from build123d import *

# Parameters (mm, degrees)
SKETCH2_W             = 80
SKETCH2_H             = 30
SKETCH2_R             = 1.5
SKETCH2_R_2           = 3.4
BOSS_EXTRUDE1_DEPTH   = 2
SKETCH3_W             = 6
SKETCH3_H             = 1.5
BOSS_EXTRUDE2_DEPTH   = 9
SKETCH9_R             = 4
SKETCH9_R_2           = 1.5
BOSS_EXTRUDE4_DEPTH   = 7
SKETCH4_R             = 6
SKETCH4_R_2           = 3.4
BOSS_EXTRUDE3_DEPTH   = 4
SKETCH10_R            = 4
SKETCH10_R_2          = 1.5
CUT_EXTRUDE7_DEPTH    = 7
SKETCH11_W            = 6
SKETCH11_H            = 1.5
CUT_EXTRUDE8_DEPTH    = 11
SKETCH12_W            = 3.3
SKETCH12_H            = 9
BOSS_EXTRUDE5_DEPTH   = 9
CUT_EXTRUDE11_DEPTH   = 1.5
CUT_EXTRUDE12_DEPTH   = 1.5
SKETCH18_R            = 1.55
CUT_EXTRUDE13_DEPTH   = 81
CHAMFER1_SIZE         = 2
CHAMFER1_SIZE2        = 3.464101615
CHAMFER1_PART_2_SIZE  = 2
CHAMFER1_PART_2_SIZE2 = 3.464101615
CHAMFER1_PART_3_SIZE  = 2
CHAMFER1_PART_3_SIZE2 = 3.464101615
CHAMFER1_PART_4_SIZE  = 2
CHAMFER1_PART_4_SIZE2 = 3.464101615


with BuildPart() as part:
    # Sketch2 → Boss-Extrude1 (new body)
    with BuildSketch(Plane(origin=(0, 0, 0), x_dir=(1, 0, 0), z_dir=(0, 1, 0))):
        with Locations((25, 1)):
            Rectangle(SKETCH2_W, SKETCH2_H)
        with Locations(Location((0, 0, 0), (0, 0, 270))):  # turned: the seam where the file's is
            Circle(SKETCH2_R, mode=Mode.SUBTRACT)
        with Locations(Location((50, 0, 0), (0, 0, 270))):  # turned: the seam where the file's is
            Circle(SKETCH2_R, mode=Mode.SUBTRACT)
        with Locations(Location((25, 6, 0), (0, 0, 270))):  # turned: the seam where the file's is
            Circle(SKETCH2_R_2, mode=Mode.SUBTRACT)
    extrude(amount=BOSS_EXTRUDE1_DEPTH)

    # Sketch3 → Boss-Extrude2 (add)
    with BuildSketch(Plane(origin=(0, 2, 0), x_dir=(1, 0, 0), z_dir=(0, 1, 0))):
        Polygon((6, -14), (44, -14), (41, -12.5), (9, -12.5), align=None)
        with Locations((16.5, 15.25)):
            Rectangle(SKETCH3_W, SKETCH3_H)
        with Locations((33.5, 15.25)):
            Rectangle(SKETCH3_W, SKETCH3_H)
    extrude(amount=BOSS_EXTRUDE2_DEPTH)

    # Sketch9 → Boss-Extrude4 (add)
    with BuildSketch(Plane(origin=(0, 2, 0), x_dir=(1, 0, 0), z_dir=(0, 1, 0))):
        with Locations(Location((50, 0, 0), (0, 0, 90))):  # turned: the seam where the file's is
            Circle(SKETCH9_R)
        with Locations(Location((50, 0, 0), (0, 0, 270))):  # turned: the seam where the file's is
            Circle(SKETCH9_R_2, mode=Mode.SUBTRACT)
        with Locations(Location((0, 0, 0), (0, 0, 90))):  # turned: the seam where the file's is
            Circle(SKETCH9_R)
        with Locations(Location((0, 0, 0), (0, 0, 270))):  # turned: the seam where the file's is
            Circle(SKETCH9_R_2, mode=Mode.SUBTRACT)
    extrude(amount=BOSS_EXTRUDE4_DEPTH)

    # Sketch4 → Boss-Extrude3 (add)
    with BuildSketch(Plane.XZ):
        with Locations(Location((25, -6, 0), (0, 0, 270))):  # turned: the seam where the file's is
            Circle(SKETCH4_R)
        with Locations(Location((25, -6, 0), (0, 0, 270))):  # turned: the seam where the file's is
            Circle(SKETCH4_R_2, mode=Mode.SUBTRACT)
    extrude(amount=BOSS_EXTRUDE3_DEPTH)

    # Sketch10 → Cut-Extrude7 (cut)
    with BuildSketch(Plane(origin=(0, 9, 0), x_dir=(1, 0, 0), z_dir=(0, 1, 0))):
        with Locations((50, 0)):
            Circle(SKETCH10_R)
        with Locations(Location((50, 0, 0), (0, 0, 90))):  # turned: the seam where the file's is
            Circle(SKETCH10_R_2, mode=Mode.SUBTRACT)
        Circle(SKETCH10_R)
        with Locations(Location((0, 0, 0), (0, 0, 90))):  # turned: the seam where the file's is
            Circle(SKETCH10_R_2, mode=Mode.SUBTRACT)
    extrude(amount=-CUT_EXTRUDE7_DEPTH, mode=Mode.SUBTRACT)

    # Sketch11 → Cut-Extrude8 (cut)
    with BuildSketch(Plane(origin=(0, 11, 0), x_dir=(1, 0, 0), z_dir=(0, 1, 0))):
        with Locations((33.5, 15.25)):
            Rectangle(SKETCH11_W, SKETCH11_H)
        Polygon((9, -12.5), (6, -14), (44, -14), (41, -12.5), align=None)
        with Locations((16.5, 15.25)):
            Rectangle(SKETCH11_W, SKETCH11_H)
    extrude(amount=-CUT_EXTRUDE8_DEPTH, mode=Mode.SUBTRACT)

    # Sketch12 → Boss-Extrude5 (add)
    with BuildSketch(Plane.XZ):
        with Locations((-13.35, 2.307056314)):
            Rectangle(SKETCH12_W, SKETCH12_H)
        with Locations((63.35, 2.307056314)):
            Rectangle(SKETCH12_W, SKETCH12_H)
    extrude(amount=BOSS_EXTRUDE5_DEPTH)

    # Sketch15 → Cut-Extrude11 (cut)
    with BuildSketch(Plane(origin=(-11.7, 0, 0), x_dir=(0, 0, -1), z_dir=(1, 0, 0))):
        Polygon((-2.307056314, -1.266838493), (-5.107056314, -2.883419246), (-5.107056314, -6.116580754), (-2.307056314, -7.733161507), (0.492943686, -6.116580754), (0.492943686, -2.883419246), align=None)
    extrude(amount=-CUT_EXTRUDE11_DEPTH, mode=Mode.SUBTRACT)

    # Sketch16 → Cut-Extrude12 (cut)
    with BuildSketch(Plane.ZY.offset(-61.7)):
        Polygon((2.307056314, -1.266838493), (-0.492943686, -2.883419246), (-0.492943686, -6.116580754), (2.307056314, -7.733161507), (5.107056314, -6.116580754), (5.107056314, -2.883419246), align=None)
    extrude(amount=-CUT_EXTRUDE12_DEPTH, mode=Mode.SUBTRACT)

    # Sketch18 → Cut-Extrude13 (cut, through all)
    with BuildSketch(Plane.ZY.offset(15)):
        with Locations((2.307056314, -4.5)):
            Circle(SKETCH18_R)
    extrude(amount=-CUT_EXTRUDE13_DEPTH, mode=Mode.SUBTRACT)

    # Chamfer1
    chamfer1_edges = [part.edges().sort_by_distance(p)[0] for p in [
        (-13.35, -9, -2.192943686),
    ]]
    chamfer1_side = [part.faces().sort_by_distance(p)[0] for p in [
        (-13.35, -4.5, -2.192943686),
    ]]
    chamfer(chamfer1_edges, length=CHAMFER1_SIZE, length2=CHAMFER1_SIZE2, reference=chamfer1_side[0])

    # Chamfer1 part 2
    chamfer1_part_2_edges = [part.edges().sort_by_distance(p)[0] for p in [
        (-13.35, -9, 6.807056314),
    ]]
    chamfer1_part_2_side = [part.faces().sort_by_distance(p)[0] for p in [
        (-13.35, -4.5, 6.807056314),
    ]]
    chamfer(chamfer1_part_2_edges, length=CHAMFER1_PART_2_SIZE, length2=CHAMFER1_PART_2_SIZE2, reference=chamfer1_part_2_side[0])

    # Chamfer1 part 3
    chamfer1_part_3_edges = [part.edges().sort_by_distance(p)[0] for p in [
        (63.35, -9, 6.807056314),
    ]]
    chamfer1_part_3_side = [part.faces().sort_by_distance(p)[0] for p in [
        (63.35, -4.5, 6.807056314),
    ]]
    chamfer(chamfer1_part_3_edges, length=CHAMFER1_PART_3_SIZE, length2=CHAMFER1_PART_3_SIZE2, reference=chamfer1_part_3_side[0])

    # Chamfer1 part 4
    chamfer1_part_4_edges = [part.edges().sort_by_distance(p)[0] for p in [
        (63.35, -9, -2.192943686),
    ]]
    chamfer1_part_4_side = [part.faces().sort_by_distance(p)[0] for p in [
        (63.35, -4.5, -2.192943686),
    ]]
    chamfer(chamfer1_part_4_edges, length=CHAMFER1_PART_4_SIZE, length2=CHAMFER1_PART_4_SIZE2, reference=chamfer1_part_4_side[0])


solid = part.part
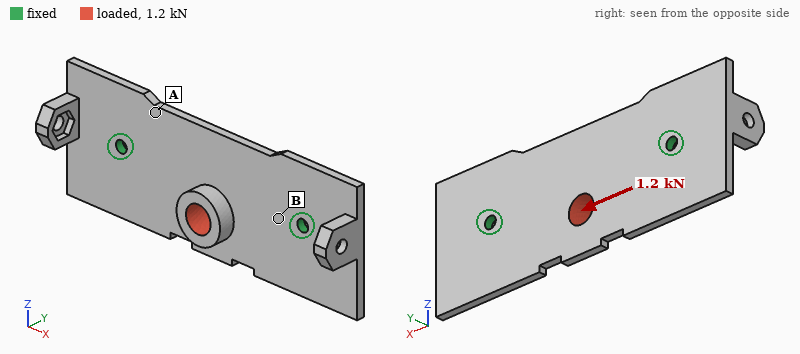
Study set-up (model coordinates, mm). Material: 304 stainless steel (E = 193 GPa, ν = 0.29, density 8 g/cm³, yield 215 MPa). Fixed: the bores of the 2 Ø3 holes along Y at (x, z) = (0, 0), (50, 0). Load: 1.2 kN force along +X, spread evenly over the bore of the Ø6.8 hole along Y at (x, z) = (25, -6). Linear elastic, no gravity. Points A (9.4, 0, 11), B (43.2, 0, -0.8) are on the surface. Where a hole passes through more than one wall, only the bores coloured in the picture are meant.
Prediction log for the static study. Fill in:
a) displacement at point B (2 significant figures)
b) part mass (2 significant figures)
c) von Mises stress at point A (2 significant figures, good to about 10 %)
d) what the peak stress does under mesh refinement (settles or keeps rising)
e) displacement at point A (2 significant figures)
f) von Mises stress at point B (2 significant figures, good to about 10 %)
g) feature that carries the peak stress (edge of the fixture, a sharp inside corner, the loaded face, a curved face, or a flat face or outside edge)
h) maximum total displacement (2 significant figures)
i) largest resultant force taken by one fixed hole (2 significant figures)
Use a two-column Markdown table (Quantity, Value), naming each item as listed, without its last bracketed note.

| Quantity | Value |
|---|---|
| displacement at point B | 3.3 µm |
| part mass | 42 g |
| von Mises stress at point A | 9.6 MPa |
| what the peak stress does under mesh refinement | keeps rising |
| displacement at point A | 2.6 µm |
| von Mises stress at point B | 25 MPa |
| feature that carries the peak stress | edge of the fixture |
| maximum total displacement | 14 µm |
| largest resultant force taken by one fixed hole | 620 N |
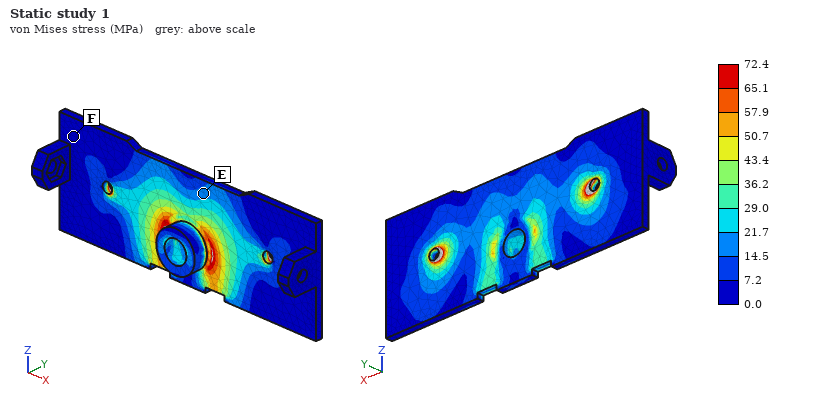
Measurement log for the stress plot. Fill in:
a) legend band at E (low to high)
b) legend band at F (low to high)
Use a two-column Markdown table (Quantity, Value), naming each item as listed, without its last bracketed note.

| Quantity | Value |
|---|---|
| legend band at E | 14.5 to 21.7 MPa |
| legend band at F | 0.0 to 7.2 MPa |
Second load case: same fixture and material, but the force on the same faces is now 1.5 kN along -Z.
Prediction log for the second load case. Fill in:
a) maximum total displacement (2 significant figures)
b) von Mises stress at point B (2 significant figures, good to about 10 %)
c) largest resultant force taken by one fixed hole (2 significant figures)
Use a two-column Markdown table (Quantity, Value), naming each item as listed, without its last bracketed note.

| Quantity | Value |
|---|---|
| maximum total displacement | 92 µm |
| von Mises stress at point B | 110 MPa |
| largest resultant force taken by one fixed hole | 760 N |
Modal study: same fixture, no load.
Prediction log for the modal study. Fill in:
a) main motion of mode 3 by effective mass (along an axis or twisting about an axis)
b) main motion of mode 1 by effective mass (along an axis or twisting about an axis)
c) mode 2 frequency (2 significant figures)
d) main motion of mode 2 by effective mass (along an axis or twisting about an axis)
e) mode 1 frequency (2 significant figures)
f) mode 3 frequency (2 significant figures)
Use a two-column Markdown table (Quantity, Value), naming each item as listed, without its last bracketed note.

| Quantity | Value |
|---|---|
| main motion of mode 3 by effective mass | twisting about Z |
| main motion of mode 1 by effective mass | along Y |
| mode 2 frequency | 3900 Hz |
| main motion of mode 2 by effective mass | twisting about X |
| mode 1 frequency | 3200 Hz |
| mode 3 frequency | 4400 Hz |
